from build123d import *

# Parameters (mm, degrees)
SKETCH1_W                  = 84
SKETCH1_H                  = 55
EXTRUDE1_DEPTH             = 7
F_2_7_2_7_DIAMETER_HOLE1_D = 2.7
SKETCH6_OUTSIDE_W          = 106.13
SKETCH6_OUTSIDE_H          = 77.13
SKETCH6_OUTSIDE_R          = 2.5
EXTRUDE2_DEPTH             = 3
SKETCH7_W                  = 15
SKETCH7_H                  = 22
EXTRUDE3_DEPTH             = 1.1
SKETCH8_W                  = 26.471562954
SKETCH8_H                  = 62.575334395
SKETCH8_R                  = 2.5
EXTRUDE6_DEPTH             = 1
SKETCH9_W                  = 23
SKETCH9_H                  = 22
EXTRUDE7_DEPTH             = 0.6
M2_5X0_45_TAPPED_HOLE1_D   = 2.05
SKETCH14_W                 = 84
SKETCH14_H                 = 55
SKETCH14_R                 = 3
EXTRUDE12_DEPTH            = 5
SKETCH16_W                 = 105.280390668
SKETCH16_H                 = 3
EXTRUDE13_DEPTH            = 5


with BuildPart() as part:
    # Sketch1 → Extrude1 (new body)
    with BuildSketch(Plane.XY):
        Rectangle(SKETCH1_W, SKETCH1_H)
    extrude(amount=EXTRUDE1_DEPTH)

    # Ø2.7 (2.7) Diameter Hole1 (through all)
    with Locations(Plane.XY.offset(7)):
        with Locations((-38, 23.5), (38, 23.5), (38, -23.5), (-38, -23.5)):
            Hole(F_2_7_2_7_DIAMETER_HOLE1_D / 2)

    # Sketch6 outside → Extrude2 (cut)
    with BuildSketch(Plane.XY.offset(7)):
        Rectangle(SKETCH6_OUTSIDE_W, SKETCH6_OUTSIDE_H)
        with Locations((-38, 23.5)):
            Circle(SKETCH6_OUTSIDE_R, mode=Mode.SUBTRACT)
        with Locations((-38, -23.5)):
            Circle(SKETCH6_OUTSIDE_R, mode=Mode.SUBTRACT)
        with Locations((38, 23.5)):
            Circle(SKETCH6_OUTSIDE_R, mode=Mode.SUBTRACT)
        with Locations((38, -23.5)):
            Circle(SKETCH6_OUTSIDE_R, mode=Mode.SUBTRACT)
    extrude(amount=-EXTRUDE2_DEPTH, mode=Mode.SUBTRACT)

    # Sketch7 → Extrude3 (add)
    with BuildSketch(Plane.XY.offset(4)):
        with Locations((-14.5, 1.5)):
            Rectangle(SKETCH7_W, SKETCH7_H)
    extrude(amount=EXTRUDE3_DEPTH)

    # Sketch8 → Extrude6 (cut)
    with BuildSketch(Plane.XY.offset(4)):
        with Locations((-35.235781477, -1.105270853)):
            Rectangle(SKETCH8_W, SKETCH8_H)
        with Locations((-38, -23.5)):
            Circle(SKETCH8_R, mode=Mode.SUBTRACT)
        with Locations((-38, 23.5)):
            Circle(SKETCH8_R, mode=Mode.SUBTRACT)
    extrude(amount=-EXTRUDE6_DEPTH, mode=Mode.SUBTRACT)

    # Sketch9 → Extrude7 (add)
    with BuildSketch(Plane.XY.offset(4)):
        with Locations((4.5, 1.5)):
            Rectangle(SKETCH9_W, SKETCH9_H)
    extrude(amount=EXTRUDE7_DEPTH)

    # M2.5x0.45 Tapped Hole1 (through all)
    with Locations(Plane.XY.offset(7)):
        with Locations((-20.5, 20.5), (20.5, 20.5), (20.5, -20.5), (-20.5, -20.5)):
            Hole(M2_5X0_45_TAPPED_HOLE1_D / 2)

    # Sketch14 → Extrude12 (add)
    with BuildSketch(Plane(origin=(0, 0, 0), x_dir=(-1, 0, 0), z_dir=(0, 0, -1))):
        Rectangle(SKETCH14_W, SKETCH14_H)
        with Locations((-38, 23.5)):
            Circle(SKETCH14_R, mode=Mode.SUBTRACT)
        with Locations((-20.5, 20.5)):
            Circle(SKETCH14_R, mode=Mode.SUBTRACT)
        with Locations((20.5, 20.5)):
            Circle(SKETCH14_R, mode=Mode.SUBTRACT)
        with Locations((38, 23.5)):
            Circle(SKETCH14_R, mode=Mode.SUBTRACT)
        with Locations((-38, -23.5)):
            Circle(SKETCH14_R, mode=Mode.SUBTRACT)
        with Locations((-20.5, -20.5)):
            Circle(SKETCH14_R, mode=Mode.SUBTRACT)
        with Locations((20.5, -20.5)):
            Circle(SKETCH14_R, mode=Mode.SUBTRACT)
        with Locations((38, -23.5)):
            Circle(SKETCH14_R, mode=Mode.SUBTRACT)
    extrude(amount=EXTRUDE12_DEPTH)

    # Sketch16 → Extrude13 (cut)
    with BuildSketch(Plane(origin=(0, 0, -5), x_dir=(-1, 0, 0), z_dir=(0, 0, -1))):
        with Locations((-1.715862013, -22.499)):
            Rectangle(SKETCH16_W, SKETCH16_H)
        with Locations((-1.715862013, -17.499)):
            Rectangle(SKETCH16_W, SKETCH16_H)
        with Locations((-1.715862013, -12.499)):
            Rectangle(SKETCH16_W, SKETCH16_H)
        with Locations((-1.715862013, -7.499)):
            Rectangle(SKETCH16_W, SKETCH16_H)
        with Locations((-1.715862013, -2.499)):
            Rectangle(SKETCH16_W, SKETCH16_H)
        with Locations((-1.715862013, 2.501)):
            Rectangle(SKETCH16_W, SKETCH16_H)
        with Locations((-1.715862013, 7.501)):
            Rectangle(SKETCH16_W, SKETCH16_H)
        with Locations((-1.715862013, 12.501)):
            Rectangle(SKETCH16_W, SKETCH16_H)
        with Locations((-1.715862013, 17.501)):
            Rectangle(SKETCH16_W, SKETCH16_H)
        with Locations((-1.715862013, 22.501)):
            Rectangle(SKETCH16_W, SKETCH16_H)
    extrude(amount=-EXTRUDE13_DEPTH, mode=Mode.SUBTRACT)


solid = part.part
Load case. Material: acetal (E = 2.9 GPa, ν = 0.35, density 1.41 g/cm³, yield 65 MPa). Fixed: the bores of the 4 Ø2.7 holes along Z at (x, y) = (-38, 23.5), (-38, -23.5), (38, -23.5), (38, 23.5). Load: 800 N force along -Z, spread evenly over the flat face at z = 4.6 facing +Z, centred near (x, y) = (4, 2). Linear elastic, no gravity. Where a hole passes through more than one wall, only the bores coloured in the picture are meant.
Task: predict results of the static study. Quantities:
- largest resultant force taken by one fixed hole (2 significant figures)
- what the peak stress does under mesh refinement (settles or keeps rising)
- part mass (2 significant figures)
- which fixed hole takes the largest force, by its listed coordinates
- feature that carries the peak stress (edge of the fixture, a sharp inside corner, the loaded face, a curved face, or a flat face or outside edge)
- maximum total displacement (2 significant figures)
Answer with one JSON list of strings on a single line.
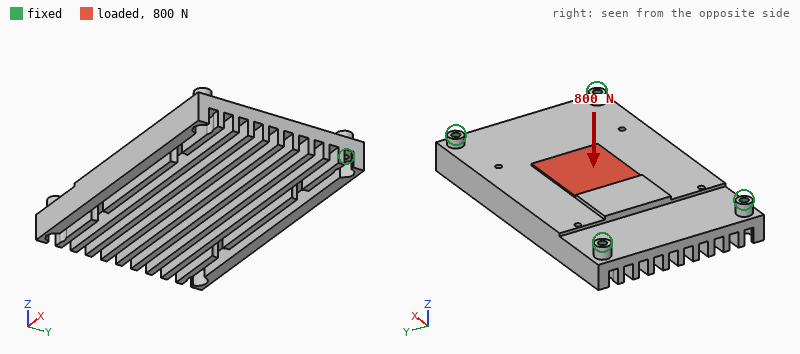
["280 N", "keeps rising", "40 g", "(38, 23.5)", "edge of the fixture", "1.1 mm"]
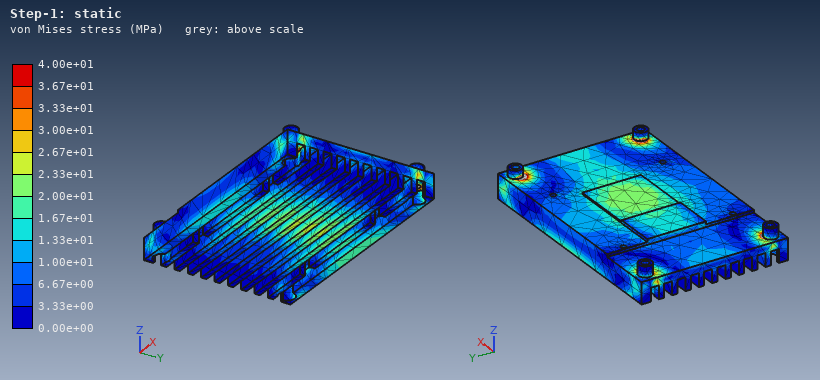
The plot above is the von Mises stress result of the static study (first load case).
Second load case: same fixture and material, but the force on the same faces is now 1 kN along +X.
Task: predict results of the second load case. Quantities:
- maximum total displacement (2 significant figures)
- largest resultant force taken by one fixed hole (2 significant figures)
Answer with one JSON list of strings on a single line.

["95 µm", "310 N"]
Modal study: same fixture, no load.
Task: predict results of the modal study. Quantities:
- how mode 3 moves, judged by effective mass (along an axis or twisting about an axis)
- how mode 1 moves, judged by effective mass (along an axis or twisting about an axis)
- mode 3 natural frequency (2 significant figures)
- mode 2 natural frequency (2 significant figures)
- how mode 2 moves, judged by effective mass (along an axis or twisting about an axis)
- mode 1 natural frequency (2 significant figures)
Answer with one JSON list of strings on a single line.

["twisting about Y", "along Z", "1900 Hz", "1600 Hz", "twisting about X", "1000 Hz"]
